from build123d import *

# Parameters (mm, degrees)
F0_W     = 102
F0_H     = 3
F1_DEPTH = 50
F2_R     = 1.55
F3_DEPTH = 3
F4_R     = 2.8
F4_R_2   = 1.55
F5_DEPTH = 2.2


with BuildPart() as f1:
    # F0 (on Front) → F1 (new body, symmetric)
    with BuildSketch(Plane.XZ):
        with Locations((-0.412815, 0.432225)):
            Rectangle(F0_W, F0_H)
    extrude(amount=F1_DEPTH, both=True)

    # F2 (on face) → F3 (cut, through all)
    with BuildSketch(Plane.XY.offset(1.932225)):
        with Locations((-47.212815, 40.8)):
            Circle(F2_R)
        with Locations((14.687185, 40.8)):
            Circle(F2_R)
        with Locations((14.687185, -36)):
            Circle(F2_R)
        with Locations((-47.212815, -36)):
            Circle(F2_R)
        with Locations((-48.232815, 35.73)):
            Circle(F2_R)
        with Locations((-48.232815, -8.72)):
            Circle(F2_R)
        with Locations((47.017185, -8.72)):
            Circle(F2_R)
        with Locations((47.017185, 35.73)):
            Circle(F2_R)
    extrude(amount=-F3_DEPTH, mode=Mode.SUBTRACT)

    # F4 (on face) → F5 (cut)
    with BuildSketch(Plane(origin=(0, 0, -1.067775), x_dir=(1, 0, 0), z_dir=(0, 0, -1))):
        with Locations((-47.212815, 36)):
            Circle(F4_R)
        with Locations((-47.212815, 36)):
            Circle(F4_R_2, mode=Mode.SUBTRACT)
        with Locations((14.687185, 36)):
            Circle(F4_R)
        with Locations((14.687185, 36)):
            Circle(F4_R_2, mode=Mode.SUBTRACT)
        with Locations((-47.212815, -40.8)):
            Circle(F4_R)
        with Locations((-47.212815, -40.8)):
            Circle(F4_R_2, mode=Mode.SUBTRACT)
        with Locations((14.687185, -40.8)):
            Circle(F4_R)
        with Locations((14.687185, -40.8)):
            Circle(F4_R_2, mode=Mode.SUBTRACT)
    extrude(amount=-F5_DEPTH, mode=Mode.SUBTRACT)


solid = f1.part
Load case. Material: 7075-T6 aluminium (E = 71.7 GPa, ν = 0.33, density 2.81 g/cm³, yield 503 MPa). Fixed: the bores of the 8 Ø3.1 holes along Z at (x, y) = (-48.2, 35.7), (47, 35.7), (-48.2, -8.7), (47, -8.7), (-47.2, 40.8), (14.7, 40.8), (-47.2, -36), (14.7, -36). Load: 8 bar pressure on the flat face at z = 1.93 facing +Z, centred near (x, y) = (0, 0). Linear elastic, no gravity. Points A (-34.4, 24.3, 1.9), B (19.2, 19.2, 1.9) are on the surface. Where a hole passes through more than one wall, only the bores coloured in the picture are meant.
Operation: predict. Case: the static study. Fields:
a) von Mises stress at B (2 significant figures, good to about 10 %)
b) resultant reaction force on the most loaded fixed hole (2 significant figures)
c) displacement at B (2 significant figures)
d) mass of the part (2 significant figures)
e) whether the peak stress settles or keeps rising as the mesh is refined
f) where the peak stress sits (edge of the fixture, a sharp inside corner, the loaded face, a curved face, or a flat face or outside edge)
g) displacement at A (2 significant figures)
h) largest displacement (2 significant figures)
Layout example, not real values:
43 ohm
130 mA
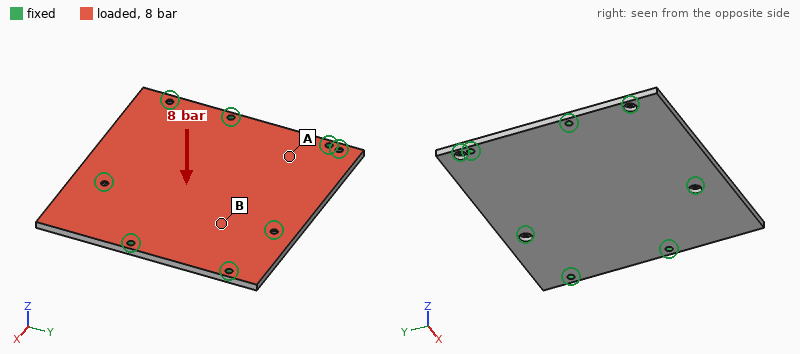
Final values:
78 MPa
2.6 kN
0.34 mm
85 g
keeps rising
edge of the fixture
0.26 mm
0.64 mm
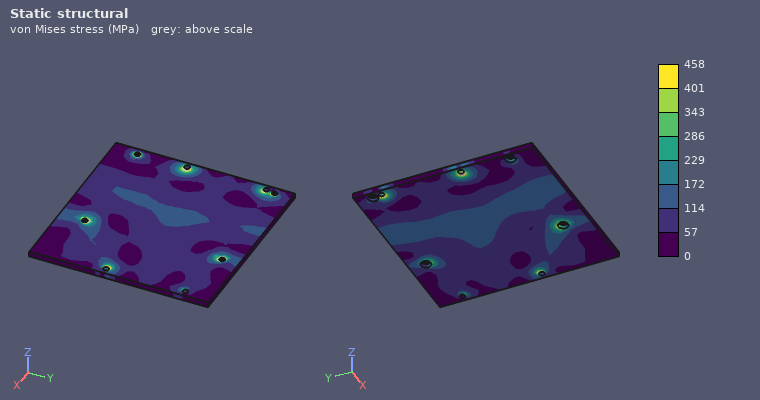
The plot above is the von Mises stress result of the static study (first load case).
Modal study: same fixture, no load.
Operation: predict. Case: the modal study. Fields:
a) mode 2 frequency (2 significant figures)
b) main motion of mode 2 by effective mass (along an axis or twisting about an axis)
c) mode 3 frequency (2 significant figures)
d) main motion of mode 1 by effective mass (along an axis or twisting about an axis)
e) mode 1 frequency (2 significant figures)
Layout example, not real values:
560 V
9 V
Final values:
2800 Hz
along Z
3300 Hz
along Z
2200 Hz
